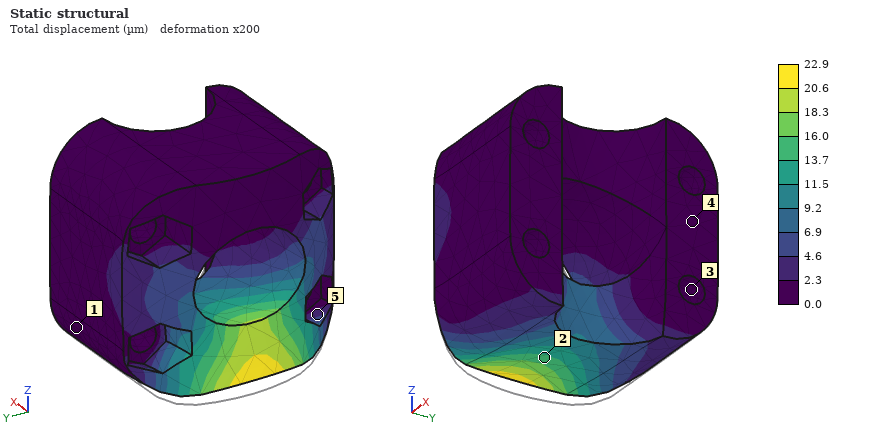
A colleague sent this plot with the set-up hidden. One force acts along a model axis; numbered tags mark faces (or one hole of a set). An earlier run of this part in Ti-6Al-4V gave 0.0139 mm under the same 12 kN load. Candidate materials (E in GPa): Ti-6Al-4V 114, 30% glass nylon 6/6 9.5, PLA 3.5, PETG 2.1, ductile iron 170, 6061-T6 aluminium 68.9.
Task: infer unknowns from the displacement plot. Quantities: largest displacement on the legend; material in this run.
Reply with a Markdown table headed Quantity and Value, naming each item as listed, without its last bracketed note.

| Quantity | Value |
|---|---|
| largest displacement on the legend | 22.9 µm |
| material in this run | 6061-T6 aluminium |
